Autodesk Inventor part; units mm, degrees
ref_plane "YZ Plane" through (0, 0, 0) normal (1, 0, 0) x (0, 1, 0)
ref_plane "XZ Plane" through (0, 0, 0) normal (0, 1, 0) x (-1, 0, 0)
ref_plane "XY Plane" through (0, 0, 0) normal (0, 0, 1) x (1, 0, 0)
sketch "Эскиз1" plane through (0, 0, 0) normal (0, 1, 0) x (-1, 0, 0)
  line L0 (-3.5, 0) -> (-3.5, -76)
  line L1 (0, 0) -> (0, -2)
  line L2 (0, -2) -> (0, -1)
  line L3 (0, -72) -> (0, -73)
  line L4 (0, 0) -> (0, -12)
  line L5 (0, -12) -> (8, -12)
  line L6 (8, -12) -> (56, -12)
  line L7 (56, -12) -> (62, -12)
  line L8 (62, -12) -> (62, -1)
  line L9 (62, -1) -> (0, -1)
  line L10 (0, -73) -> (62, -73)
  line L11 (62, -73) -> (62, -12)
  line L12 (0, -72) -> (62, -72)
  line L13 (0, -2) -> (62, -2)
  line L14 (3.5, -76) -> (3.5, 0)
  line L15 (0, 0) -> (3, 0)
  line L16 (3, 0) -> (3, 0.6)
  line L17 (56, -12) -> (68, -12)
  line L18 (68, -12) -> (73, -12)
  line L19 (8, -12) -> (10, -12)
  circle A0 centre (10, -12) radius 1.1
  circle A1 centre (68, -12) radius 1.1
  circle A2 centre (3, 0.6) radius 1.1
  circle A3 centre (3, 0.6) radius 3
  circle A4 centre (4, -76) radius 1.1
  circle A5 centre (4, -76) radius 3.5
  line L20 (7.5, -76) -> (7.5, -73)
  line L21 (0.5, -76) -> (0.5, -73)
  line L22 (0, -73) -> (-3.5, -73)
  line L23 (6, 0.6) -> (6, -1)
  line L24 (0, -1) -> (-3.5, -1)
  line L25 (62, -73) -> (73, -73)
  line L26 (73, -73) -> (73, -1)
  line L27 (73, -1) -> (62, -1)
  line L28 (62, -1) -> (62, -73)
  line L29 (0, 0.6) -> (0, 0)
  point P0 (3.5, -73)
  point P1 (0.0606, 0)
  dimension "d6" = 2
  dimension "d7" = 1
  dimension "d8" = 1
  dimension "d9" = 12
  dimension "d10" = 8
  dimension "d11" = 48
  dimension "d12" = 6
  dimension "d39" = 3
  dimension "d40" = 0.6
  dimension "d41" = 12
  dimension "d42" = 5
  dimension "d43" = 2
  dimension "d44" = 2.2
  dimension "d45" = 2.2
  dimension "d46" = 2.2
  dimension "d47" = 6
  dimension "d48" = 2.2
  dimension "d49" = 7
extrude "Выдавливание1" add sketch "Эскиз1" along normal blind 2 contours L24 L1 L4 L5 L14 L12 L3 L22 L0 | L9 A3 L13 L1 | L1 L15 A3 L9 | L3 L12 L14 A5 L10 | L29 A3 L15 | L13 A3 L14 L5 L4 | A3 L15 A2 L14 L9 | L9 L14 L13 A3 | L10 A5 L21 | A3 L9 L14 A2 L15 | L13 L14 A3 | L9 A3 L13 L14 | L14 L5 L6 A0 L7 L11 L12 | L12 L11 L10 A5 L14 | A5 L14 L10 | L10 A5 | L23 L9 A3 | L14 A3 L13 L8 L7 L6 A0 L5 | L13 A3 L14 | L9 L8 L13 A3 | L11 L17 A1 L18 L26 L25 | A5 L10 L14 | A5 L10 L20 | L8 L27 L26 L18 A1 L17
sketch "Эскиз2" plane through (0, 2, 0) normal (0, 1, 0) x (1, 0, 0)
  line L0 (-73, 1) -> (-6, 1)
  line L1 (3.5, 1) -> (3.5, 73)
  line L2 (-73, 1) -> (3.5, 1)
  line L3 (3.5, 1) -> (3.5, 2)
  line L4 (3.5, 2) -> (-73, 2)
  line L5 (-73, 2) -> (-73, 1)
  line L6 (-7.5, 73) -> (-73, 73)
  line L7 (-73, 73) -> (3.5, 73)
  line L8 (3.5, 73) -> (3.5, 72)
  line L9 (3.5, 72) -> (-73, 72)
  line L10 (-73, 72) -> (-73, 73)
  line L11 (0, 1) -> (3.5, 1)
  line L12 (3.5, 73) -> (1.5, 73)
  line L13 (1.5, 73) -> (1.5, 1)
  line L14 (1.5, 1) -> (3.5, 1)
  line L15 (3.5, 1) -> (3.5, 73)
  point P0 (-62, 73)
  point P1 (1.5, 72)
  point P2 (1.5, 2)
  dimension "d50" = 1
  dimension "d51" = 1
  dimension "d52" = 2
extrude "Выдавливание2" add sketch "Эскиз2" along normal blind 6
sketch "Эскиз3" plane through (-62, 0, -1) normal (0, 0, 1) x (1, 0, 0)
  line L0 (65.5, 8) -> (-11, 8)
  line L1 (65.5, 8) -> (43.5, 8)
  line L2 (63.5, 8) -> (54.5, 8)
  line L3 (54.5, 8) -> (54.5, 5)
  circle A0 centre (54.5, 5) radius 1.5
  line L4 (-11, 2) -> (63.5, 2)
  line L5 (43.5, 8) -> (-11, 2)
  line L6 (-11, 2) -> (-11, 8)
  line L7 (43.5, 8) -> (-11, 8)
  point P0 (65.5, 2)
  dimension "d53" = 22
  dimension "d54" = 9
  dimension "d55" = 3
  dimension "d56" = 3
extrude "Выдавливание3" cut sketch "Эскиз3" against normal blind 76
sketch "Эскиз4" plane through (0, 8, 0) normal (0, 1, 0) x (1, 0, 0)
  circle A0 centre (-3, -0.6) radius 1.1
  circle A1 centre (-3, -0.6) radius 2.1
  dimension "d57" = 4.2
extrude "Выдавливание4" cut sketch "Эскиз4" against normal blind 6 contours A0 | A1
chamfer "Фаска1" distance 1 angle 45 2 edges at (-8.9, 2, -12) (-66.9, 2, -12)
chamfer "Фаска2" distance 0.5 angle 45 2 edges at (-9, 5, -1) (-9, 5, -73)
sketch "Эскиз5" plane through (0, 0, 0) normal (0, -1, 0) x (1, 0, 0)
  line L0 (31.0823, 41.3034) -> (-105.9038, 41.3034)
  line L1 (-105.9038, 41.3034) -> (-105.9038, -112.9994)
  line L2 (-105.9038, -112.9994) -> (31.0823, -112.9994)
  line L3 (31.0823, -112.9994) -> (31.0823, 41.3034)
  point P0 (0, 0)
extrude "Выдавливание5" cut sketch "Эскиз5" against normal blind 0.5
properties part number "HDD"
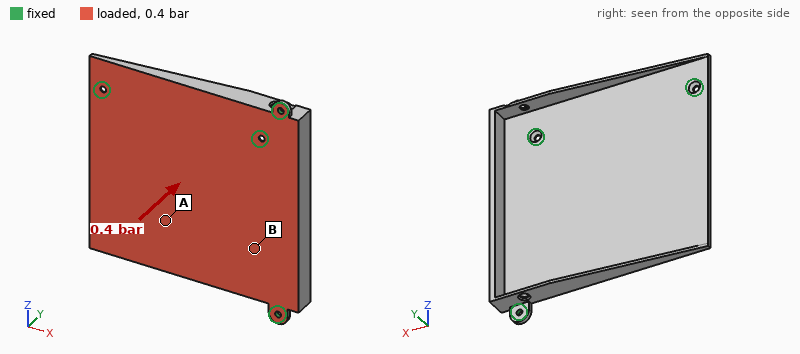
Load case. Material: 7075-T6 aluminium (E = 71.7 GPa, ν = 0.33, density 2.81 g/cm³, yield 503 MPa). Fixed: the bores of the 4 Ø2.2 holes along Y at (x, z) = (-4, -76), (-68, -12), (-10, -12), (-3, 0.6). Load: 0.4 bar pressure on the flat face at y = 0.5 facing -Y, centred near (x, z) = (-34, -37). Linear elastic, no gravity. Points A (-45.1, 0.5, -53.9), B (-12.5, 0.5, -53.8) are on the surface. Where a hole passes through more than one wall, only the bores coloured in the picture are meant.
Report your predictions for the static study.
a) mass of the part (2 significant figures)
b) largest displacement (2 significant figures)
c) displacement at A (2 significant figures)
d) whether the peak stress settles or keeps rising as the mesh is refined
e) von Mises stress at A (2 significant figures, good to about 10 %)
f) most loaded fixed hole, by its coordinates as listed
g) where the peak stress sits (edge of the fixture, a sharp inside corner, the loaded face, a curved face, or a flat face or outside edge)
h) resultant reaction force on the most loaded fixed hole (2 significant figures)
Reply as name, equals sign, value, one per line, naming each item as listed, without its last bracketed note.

mass of the part = 27 g
largest displacement = 1.3 mm
displacement at A = 0.63 mm
whether the peak stress settles or keeps rising as the mesh is refined = keeps rising
von Mises stress at A = 34 MPa
most loaded fixed hole, by its coordinates as listed = (-10, -12)
where the peak stress sits = edge of the fixture
resultant reaction force on the most loaded fixed hole = 160 N
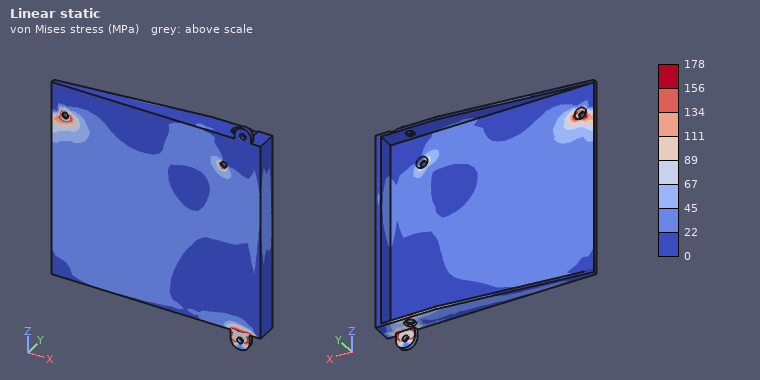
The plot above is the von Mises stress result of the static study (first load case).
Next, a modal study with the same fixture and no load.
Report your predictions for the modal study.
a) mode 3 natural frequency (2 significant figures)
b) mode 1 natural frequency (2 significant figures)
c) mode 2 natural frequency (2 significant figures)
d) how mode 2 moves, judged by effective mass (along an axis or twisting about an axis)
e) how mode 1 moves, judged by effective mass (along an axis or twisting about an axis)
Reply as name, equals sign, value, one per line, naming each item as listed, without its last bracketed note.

mode 3 natural frequency = 2100 Hz
mode 1 natural frequency = 600 Hz
mode 2 natural frequency = 1800 Hz
how mode 2 moves, judged by effective mass = along Y
how mode 1 moves, judged by effective mass = along Y
